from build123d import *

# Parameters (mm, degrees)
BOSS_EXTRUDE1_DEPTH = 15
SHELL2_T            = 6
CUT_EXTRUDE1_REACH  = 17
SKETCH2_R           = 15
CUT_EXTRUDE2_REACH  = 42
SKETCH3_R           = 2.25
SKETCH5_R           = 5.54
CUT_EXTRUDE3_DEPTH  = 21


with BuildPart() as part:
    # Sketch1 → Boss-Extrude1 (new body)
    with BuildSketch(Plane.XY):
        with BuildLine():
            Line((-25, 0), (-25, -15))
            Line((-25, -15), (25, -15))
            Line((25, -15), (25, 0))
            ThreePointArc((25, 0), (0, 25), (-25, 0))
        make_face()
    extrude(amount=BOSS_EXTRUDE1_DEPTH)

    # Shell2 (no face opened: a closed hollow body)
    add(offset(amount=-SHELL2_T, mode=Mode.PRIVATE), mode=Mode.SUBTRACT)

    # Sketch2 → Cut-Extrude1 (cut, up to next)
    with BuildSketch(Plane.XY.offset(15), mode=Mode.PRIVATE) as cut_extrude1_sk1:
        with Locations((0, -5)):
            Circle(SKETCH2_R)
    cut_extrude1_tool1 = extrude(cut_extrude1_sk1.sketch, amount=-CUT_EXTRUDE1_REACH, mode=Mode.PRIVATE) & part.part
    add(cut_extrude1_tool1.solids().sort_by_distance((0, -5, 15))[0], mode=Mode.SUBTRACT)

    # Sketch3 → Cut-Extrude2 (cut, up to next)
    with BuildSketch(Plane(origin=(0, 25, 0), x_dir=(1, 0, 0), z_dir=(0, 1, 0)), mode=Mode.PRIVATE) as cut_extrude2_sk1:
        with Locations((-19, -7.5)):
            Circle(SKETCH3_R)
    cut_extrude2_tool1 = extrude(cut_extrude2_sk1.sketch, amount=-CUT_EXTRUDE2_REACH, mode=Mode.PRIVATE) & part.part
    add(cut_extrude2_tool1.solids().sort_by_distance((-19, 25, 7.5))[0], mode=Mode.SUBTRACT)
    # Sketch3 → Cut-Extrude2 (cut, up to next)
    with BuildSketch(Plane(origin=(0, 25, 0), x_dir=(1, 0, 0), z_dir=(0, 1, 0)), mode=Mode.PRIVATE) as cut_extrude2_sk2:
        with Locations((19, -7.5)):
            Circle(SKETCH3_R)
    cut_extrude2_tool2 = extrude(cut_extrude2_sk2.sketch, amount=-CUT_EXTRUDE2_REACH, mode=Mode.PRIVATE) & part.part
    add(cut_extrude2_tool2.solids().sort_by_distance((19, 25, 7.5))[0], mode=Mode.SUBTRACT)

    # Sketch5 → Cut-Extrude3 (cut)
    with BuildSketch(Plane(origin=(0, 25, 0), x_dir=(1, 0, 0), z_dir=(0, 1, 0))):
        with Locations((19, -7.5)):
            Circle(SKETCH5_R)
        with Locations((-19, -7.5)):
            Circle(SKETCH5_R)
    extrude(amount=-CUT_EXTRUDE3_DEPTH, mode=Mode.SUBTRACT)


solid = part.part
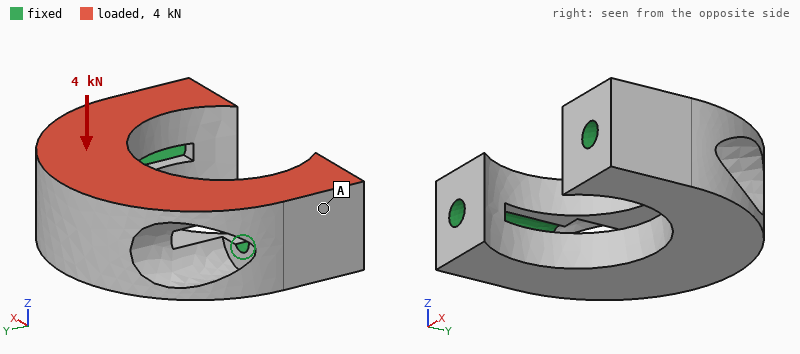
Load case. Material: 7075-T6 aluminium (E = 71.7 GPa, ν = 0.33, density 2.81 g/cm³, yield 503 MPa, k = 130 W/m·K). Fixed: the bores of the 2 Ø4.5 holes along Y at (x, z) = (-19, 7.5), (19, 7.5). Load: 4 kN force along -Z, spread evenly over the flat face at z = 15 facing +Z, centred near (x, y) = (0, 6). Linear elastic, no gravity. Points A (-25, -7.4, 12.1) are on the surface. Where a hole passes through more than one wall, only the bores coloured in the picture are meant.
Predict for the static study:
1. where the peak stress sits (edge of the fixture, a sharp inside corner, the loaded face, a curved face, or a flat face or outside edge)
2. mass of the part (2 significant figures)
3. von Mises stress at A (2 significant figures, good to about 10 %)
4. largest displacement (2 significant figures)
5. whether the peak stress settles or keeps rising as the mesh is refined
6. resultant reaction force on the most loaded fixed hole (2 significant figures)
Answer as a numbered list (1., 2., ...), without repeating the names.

1. edge of the fixture
2. 36 g
3. 16 MPa
4. 69 µm
5. keeps rising
6. 2.0 kN
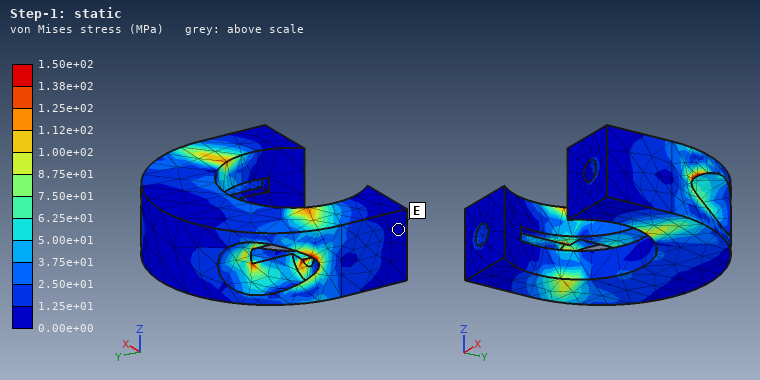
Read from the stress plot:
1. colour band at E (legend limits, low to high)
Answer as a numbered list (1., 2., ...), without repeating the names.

1. 0.00e+00 to 1.25e+01 MPa
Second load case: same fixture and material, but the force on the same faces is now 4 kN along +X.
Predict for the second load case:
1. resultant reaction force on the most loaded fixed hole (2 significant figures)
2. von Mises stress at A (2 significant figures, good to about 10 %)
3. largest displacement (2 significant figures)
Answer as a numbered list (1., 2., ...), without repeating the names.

1. 2.1 kN
2. 11 MPa
3. 26 µm
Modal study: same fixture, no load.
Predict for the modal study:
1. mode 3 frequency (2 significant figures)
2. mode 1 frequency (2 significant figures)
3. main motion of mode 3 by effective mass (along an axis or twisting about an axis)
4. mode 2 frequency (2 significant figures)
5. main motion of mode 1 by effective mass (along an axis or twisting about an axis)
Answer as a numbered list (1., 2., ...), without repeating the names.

1. 18 kHz
2. 7300 Hz
3. along X
4. 17 kHz
5. along Z
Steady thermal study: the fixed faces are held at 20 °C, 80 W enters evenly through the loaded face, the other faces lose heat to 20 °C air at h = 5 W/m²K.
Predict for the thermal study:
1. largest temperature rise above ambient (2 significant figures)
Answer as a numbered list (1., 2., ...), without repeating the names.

1. 37 K
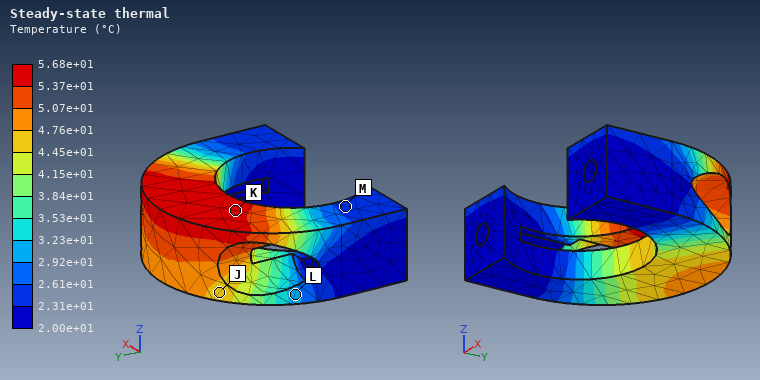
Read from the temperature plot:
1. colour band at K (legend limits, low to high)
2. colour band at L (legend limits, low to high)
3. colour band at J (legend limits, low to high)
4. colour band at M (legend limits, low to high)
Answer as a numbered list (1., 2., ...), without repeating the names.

1. 5.37e+01 to 5.68e+01 °C
2. 2.92e+01 to 3.23e+01 °C
3. 4.45e+01 to 4.76e+01 °C
4. 2.31e+01 to 2.61e+01 °C
